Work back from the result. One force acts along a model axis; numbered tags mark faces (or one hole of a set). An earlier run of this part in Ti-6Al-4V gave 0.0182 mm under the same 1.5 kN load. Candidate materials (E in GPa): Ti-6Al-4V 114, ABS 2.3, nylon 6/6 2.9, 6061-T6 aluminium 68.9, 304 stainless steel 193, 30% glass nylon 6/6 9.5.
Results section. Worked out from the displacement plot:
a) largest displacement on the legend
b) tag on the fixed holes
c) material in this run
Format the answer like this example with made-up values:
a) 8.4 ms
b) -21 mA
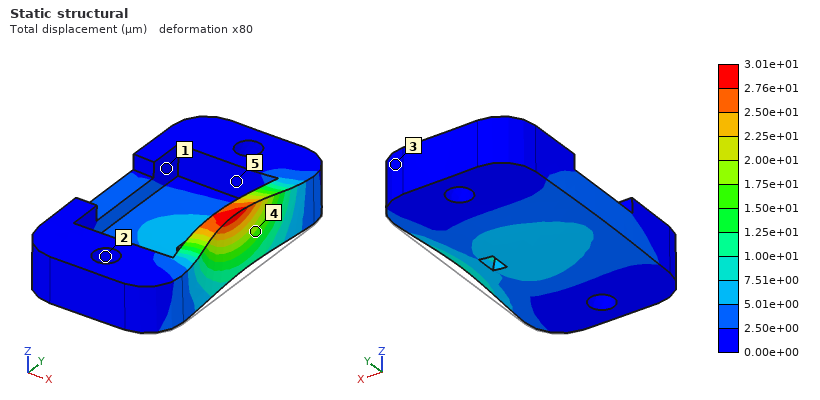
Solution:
a) 3.01e+01 µm
b) 2
c) 6061-T6 aluminium
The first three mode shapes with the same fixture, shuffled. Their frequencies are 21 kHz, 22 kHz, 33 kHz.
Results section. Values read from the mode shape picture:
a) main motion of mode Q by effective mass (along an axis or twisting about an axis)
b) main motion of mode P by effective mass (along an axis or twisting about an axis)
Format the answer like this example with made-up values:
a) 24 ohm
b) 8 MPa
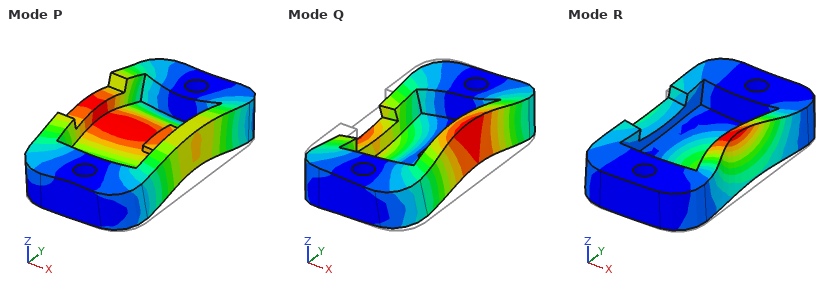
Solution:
a) twisting about Y
b) along Z
